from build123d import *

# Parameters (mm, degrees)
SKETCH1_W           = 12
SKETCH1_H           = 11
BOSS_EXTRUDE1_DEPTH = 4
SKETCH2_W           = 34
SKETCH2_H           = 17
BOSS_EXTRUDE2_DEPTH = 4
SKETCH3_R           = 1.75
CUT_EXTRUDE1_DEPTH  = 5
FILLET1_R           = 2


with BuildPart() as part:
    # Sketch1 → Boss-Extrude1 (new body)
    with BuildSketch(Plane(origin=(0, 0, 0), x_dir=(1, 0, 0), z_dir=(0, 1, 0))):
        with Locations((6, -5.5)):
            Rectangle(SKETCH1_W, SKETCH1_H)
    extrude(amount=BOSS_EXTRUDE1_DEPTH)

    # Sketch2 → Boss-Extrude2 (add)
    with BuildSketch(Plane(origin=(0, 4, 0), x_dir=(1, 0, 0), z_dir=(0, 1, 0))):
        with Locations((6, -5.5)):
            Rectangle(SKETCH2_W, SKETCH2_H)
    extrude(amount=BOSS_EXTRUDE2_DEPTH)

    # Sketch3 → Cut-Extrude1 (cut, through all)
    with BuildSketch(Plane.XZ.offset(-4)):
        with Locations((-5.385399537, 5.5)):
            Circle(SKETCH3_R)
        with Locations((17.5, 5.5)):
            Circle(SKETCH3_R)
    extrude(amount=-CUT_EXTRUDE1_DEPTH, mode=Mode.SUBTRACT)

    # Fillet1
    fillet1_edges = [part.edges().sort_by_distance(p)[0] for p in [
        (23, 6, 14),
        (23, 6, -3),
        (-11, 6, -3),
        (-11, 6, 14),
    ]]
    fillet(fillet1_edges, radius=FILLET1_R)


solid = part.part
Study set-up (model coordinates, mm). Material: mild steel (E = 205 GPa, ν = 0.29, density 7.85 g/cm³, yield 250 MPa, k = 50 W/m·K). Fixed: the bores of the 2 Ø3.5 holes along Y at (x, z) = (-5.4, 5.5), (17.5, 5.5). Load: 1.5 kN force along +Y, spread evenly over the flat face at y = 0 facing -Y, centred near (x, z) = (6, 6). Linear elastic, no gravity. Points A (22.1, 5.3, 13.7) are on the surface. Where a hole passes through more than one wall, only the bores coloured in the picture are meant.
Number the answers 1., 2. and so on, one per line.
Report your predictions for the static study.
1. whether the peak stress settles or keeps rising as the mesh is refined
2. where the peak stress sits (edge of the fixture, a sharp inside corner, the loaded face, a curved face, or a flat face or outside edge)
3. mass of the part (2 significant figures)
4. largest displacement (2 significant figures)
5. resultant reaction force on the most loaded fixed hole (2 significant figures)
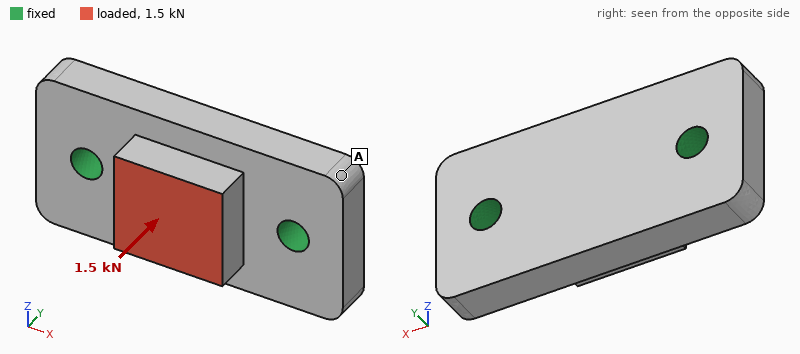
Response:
1. keeps rising
2. edge of the fixture
3. 22 g
4. 3.7 µm
5. 790 N
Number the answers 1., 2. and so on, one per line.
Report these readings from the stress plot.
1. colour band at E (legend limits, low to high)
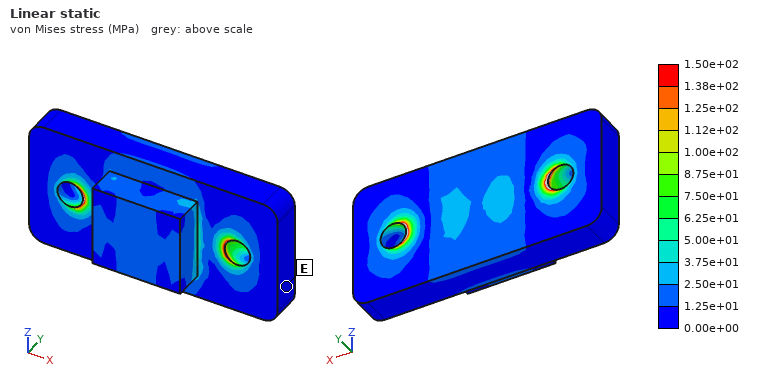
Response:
1. 0.00e+00 to 1.25e+01 MPa
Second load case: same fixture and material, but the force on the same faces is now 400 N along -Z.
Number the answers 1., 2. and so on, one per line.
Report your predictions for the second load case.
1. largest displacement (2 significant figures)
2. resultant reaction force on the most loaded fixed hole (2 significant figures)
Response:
1. 2.9 µm
2. 200 N
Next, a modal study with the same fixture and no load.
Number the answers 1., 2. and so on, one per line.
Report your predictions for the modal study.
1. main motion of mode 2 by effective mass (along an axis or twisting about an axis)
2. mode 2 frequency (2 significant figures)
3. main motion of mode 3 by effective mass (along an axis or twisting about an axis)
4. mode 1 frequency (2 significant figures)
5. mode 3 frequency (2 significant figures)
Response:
1. along Y
2. 31 kHz
3. along Z
4. 25 kHz
5. 45 kHz
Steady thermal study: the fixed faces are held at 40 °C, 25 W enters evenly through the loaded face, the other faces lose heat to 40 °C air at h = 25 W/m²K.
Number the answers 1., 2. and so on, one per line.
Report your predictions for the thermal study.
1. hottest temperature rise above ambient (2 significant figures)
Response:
1. 49 K
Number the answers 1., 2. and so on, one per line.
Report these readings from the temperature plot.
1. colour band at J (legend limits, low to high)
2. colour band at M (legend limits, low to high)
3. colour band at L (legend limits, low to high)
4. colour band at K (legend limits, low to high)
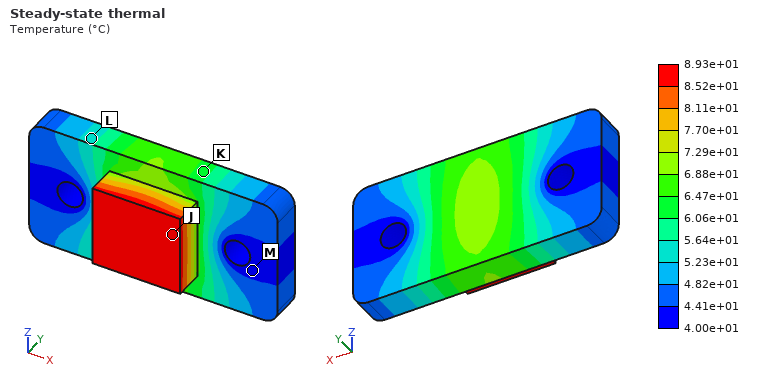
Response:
1. 8.52e+01 to 8.93e+01 °C
2. 4.00e+01 to 4.41e+01 °C
3. 5.23e+01 to 5.64e+01 °C
4. 6.06e+01 to 6.47e+01 °C
